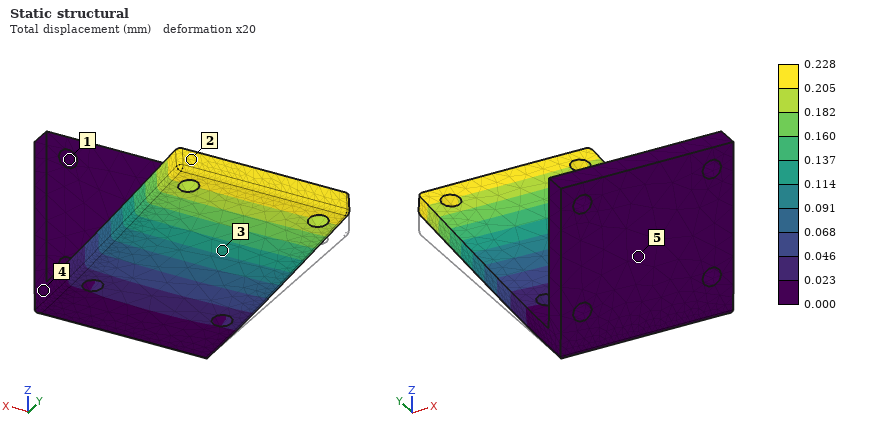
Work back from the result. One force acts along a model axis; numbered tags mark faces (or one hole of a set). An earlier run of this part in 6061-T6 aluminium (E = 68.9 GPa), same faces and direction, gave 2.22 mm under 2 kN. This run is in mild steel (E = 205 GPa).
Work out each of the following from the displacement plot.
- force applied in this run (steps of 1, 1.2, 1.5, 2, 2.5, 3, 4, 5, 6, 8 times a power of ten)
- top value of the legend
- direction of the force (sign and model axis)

600 N
0.228 mm
+Z
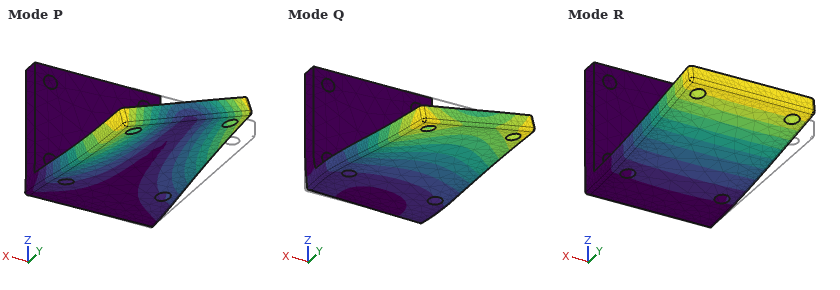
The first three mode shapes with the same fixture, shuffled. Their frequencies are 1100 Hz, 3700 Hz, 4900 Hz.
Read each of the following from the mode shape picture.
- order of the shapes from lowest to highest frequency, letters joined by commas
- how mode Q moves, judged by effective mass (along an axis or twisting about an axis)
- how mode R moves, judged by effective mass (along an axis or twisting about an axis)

R, P, Q
along X
along Z
